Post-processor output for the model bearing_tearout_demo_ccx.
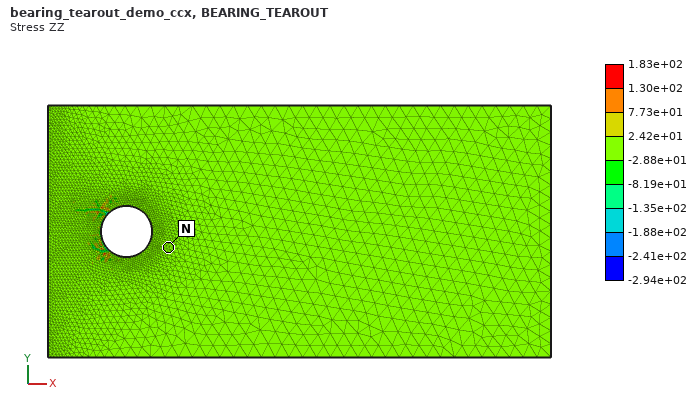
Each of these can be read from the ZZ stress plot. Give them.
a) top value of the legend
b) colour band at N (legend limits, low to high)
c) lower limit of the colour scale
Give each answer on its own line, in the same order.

1.83e+02
-2.88e+01 to 2.42e+01
-2.94e+02
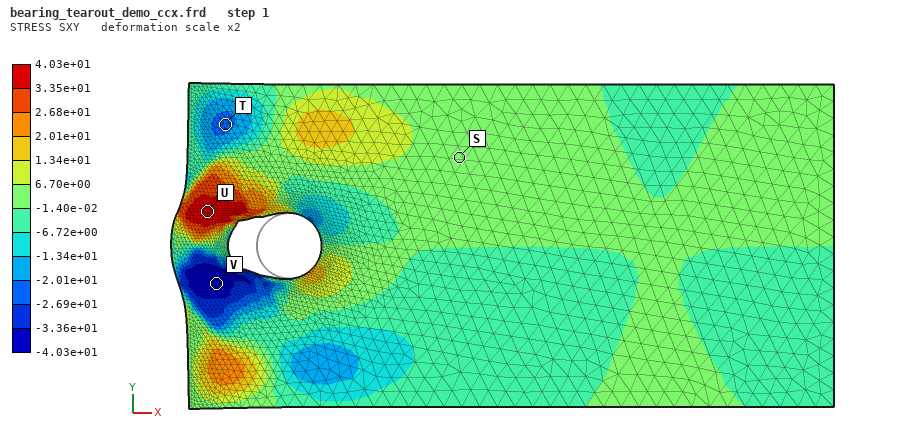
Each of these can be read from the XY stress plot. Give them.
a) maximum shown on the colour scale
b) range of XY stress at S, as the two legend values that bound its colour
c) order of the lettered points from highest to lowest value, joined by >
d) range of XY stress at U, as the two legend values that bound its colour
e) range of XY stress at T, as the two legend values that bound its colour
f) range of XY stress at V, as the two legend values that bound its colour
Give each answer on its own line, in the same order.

4.03e+01
-1.40e-02 to 6.70e+00
U > S > T > V
3.35e+01 to 4.03e+01
-2.69e+01 to -2.01e+01
-4.03e+01 to -3.36e+01
